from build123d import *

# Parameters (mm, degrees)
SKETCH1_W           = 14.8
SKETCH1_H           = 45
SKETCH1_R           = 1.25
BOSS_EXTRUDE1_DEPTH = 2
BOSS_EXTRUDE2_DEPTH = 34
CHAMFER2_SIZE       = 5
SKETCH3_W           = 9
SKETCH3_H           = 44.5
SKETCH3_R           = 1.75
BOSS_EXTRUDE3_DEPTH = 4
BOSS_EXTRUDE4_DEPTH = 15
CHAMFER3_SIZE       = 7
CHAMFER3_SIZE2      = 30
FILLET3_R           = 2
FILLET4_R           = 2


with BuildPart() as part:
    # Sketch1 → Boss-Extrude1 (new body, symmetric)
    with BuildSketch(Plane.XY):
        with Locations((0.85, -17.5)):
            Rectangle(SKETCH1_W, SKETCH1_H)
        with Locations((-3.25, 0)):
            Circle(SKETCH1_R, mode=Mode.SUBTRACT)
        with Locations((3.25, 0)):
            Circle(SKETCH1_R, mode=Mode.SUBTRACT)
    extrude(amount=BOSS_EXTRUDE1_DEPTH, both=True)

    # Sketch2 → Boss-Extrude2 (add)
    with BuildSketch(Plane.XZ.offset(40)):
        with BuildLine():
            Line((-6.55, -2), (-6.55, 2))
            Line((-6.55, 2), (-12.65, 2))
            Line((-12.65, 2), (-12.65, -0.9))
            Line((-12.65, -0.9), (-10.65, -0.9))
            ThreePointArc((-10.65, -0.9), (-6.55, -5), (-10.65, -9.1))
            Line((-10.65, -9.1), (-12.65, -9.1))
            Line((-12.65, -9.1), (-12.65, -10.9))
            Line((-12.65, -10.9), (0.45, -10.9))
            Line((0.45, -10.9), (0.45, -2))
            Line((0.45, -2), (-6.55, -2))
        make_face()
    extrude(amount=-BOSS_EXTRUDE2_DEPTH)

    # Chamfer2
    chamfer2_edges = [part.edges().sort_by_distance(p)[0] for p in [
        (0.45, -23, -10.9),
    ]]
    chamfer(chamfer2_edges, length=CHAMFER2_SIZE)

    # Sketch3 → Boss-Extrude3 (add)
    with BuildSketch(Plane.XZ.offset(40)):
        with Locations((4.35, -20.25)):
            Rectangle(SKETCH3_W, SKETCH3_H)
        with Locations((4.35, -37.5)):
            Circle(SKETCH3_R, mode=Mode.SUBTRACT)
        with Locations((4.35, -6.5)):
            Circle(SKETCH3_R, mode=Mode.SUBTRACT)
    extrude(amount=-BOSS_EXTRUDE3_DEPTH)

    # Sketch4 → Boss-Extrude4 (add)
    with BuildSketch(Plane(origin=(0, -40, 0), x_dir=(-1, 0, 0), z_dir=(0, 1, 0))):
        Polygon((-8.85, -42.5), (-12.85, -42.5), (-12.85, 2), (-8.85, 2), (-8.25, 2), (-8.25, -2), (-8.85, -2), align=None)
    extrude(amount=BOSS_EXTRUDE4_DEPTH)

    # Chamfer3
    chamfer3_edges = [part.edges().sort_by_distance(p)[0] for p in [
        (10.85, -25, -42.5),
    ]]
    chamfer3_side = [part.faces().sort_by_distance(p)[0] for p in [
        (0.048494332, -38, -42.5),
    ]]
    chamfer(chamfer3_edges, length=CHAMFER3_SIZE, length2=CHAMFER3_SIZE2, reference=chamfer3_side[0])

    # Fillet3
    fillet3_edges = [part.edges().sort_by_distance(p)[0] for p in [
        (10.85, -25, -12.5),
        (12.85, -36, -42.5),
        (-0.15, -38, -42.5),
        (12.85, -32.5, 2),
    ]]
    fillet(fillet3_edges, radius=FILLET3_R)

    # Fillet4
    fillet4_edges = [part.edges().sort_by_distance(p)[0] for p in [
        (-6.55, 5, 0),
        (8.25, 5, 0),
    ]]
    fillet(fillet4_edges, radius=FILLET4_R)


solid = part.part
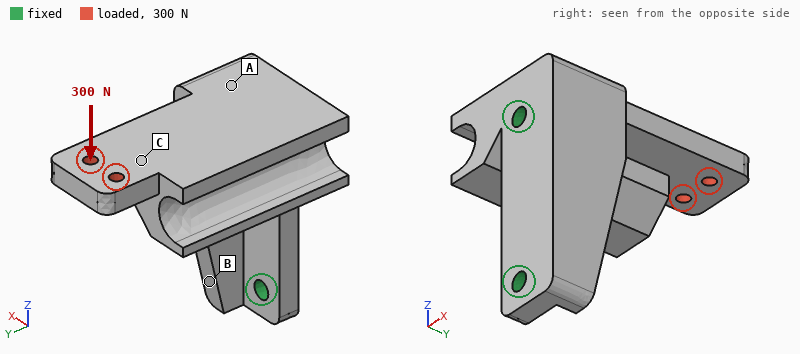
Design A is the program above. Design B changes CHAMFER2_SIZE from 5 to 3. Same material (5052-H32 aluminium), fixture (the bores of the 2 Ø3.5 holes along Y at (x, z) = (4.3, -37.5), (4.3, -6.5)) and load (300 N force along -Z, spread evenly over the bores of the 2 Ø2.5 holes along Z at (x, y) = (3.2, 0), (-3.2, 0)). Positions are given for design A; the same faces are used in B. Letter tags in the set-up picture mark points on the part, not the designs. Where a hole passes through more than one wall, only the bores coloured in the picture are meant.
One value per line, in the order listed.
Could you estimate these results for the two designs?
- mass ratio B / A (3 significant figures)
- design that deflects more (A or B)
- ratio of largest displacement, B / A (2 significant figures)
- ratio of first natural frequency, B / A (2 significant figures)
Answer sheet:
1.03
A
0.81
1.0
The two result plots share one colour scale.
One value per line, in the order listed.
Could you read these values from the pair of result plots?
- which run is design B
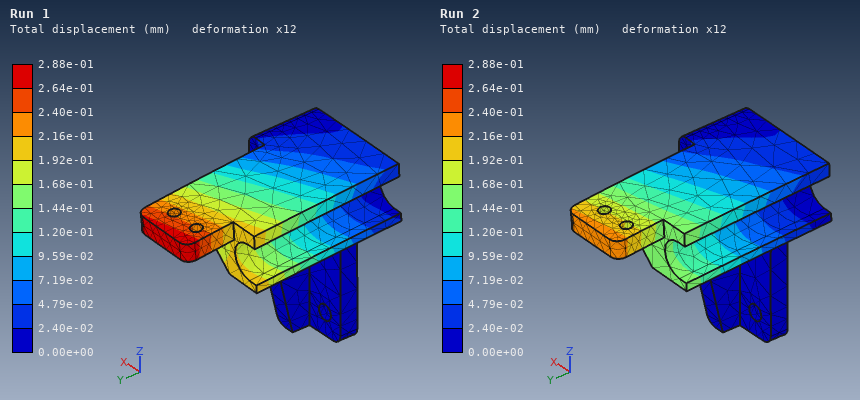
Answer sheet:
Run 2
